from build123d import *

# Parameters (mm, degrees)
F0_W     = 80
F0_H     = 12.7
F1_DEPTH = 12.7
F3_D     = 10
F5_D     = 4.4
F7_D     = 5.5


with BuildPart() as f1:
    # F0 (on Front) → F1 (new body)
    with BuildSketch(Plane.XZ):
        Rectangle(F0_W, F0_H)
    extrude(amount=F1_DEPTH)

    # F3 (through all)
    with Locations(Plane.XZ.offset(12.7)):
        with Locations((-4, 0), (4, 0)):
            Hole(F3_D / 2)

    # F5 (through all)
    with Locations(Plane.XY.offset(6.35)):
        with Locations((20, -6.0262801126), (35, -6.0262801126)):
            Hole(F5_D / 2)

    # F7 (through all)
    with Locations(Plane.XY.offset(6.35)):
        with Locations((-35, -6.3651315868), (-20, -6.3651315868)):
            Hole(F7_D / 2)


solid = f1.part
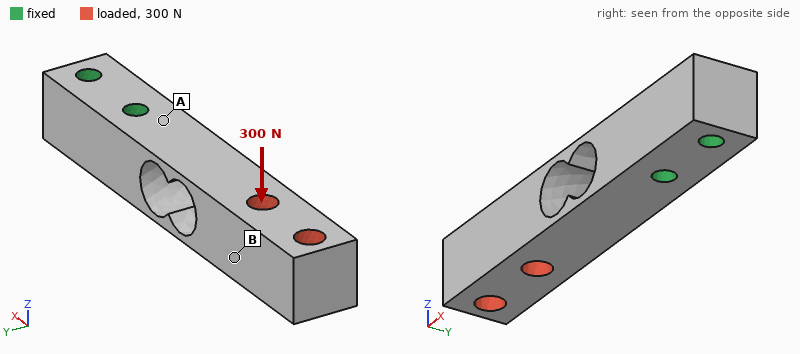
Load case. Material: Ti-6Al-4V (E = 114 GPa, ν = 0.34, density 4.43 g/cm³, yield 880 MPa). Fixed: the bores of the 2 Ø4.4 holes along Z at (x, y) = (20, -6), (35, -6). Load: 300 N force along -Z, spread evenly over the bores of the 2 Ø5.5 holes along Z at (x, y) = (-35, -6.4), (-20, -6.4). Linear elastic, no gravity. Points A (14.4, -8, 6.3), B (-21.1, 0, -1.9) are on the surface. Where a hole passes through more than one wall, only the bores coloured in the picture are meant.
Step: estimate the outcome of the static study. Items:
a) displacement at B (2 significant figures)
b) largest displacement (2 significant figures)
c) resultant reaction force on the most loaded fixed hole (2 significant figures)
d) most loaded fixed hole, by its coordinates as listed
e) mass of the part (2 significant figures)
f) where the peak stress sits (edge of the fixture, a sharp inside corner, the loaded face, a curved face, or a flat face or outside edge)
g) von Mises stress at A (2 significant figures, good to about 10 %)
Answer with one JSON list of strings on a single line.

["0.13 mm", "0.17 mm", "410 N", "(20, -6)", "44 g", "a curved face", "46 MPa"]
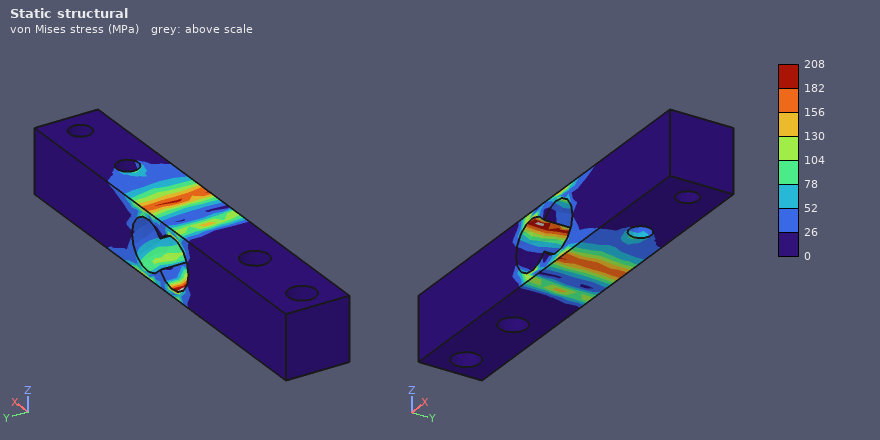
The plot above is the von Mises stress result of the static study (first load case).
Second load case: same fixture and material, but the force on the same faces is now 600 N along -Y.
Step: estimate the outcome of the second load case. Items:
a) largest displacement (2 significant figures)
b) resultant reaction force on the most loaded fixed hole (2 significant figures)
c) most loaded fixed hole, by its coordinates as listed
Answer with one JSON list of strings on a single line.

["0.33 mm", "1.4 kN", "(20, -6)"]
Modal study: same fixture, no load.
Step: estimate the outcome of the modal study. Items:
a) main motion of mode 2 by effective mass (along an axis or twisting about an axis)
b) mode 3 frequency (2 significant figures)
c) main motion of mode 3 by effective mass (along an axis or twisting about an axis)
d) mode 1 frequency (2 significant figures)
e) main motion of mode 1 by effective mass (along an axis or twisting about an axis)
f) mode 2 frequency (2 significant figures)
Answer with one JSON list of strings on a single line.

["along Y", "6900 Hz", "twisting about X", "1700 Hz", "along Z", "1900 Hz"]
